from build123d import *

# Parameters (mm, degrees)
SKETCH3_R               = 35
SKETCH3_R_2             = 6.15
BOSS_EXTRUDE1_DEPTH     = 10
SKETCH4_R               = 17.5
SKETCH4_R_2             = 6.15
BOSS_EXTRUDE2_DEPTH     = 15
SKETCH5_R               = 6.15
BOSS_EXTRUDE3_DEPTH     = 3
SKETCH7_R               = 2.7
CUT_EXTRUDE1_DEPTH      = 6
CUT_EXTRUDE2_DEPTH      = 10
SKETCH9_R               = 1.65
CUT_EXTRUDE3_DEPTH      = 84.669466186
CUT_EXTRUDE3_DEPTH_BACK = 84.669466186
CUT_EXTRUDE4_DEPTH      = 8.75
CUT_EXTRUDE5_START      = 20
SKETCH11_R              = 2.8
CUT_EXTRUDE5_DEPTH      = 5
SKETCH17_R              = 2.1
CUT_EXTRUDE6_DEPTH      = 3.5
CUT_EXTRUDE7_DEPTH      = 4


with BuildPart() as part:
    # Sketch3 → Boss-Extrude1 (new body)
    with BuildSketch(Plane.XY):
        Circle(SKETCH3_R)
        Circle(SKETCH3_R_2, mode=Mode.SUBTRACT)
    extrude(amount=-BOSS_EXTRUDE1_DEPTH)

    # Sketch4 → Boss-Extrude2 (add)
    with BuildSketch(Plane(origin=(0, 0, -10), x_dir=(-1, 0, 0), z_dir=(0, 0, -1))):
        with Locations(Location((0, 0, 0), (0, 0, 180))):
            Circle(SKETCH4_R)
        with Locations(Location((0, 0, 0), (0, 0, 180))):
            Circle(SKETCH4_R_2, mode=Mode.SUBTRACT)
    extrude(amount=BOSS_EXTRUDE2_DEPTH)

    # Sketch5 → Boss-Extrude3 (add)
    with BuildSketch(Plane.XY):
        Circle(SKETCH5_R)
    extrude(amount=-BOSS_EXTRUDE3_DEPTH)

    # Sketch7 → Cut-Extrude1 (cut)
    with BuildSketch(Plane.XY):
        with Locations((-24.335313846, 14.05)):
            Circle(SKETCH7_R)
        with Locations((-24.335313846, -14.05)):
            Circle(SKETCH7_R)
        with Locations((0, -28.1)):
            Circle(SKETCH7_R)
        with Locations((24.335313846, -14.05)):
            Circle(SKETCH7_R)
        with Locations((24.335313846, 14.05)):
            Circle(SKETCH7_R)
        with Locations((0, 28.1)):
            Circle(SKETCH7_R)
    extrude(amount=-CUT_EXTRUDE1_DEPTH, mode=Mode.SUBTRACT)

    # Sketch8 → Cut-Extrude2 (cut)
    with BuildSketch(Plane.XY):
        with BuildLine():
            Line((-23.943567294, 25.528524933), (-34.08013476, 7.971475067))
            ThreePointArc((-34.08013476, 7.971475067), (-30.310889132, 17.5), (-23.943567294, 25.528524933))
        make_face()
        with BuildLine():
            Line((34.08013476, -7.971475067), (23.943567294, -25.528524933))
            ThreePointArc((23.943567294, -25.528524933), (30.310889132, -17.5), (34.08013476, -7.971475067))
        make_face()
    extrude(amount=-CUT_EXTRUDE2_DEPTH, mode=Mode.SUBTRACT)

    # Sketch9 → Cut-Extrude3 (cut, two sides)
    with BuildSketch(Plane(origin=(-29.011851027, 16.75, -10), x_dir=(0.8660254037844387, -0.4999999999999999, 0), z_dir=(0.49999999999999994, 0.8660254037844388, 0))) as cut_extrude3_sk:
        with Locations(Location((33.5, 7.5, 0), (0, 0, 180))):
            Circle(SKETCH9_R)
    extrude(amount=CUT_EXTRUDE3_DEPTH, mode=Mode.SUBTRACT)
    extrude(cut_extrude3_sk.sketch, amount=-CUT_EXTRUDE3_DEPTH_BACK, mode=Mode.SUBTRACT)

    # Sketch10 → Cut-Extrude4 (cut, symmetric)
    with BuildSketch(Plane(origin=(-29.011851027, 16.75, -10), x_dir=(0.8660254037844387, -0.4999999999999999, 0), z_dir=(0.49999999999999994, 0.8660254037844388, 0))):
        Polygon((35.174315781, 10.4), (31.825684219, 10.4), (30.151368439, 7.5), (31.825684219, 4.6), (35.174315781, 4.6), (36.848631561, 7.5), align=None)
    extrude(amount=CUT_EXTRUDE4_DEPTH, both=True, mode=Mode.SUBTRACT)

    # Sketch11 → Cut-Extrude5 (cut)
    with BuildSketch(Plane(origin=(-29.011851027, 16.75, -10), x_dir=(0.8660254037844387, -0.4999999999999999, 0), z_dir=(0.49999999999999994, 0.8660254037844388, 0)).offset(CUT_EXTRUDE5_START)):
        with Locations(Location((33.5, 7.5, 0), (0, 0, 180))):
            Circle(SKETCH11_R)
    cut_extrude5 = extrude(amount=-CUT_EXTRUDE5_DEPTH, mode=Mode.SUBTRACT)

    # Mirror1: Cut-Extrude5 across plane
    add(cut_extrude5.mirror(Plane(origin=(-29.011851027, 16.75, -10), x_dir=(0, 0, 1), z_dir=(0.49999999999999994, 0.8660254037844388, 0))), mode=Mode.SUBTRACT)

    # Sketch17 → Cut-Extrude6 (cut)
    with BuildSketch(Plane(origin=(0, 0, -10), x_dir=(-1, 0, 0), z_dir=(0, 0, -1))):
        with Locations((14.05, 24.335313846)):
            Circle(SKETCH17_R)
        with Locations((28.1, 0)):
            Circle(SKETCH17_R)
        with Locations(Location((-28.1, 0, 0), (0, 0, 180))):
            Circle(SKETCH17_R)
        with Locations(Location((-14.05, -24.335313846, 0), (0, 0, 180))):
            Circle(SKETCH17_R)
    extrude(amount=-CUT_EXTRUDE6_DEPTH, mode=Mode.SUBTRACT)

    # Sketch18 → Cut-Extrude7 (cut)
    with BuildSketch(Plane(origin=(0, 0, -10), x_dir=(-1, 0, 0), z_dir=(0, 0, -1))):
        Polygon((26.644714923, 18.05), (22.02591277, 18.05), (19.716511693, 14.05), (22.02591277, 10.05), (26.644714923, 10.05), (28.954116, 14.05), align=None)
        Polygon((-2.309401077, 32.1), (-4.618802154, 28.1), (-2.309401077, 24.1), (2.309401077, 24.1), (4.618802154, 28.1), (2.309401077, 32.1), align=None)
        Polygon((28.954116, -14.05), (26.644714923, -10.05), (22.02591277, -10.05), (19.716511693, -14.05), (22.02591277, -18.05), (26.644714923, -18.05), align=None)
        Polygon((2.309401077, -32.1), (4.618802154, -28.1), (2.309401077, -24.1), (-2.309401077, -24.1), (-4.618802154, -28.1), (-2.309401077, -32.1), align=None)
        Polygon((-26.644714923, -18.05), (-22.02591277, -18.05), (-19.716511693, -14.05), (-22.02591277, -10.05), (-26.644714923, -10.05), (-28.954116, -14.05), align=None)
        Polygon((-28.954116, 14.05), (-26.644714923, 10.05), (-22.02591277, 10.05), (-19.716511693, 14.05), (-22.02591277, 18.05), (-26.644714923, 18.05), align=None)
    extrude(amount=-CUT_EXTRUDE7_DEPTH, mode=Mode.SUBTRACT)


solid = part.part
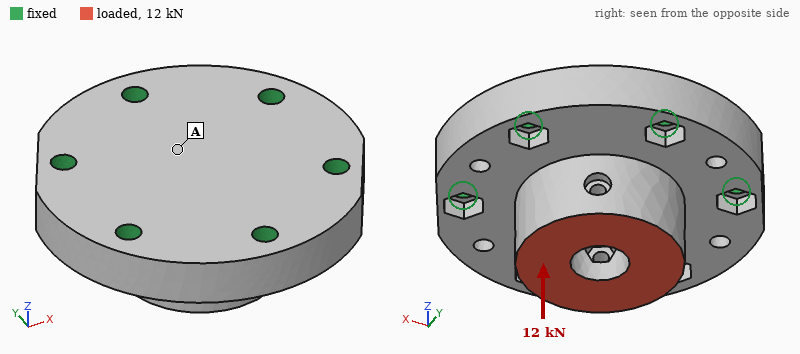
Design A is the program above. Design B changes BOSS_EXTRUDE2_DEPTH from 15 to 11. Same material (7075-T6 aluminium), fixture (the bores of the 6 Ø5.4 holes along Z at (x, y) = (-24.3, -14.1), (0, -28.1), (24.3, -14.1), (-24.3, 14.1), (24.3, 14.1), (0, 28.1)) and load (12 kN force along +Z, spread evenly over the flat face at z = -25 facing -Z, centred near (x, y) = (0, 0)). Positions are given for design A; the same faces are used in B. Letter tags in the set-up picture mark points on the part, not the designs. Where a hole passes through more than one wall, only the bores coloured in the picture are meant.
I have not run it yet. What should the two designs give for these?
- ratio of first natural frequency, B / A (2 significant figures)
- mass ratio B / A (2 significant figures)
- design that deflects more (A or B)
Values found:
1.1
0.93
B
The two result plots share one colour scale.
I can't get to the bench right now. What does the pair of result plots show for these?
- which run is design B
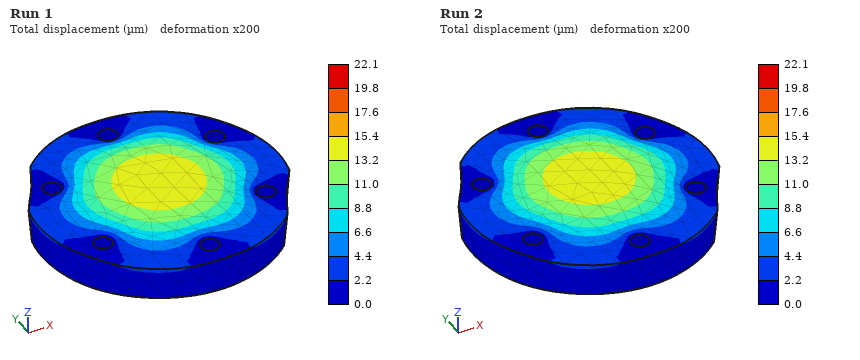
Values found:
Run 1
